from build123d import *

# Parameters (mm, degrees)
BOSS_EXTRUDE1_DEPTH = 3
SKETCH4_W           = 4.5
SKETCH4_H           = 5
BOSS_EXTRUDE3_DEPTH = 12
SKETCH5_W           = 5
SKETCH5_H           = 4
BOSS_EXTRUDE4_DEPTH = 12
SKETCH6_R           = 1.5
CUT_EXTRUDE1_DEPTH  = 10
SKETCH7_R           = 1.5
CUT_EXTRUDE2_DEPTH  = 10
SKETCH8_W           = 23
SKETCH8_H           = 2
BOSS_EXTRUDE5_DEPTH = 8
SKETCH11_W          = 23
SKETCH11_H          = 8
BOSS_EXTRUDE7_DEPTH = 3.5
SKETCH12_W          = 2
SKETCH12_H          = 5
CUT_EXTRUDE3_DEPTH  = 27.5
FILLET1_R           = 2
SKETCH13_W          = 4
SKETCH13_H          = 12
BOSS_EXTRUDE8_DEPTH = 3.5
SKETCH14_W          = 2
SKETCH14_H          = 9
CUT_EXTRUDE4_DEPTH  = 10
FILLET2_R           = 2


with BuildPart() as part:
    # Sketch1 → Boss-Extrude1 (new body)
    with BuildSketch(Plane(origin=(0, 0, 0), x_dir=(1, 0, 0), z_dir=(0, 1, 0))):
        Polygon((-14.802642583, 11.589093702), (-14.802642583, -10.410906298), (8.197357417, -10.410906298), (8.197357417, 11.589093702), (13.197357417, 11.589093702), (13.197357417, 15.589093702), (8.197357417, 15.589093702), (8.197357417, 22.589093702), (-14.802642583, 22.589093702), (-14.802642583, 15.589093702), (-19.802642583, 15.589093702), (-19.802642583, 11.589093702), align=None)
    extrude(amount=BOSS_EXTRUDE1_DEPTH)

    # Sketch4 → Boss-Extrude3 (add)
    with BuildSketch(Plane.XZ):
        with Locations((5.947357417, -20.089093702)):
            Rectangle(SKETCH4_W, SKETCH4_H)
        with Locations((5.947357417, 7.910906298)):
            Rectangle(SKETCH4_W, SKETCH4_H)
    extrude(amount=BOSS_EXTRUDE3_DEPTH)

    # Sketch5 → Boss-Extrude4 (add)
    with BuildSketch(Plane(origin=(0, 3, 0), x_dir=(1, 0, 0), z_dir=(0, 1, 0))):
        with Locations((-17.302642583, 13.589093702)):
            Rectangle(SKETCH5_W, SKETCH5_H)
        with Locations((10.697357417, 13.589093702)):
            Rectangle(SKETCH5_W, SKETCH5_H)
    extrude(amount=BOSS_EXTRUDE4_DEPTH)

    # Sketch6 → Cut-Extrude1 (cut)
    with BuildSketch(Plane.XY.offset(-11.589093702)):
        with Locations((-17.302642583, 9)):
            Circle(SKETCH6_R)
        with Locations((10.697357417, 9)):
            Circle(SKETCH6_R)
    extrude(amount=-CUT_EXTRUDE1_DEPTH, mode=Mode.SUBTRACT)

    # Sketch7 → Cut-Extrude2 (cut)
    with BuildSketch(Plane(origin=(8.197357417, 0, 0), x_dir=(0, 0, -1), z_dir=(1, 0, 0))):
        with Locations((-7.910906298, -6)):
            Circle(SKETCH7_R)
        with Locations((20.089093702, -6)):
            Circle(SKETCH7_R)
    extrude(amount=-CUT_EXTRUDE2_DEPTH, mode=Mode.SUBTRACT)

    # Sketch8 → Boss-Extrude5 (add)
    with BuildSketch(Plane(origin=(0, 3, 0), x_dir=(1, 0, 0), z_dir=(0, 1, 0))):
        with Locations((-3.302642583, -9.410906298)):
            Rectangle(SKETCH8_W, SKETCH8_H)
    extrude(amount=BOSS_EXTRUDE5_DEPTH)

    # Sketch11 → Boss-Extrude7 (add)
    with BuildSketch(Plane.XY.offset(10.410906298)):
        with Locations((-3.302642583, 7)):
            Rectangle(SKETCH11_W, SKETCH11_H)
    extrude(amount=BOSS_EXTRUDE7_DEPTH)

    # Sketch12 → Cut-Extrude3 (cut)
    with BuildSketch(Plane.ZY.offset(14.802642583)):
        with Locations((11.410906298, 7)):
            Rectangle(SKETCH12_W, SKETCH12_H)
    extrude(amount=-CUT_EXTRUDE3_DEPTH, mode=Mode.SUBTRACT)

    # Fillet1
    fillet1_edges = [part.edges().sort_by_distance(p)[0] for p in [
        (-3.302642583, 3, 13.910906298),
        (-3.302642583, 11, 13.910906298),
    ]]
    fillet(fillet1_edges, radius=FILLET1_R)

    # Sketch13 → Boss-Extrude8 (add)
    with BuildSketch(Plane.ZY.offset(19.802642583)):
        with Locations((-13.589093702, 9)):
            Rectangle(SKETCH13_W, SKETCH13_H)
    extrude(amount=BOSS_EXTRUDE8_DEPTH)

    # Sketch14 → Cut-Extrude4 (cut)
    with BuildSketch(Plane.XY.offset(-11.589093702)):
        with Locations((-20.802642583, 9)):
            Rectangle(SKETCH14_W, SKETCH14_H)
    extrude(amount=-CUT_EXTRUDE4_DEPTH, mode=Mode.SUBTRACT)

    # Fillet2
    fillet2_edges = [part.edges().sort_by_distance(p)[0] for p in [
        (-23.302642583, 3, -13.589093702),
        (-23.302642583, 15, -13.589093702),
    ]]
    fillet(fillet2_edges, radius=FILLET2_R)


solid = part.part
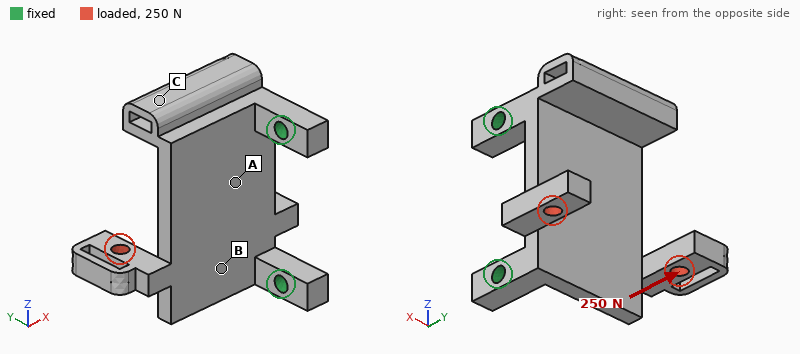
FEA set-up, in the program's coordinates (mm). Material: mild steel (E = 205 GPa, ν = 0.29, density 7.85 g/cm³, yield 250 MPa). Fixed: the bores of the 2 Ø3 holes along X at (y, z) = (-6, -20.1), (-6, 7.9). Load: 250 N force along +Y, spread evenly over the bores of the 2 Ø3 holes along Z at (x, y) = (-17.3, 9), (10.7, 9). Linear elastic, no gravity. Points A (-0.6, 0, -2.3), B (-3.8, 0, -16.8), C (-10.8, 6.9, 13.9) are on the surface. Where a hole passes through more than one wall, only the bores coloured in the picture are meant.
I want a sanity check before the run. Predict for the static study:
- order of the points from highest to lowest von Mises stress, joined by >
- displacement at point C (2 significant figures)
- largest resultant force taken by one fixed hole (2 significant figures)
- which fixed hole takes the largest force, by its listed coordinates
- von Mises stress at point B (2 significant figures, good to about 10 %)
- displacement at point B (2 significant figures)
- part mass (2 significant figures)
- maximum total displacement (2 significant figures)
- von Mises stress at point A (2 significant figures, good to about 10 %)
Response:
B > A > C
0.021 mm
220 N
(-6, -20.1)
42 MPa
0.018 mm
32 g
0.10 mm
22 MPa
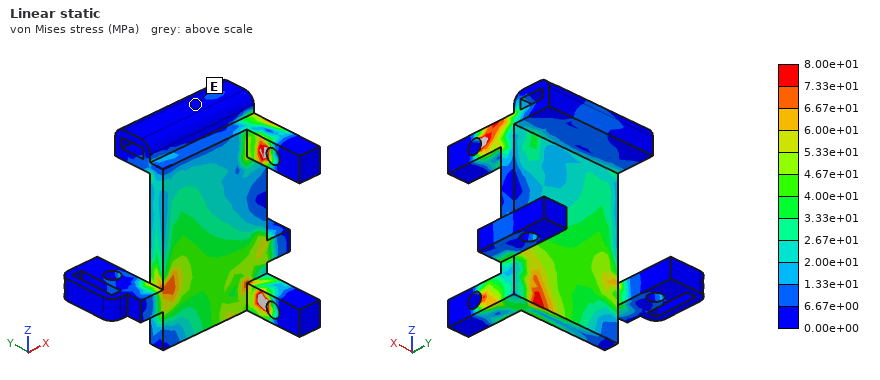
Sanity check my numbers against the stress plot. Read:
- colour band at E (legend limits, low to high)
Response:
0.00e+00 to 6.67e+00 MPa
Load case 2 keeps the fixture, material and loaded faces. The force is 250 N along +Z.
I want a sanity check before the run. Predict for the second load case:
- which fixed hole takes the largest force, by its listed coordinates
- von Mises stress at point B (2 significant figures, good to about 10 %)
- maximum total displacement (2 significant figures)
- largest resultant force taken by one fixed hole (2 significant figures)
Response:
(-6, 7.9)
17 MPa
38 µm
200 N
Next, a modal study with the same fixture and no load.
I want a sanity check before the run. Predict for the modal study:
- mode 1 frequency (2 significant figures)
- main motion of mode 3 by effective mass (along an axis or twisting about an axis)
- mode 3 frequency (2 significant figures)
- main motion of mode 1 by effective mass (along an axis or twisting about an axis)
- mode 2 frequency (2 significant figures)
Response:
2400 Hz
along Z
6900 Hz
along Y
5000 Hz
